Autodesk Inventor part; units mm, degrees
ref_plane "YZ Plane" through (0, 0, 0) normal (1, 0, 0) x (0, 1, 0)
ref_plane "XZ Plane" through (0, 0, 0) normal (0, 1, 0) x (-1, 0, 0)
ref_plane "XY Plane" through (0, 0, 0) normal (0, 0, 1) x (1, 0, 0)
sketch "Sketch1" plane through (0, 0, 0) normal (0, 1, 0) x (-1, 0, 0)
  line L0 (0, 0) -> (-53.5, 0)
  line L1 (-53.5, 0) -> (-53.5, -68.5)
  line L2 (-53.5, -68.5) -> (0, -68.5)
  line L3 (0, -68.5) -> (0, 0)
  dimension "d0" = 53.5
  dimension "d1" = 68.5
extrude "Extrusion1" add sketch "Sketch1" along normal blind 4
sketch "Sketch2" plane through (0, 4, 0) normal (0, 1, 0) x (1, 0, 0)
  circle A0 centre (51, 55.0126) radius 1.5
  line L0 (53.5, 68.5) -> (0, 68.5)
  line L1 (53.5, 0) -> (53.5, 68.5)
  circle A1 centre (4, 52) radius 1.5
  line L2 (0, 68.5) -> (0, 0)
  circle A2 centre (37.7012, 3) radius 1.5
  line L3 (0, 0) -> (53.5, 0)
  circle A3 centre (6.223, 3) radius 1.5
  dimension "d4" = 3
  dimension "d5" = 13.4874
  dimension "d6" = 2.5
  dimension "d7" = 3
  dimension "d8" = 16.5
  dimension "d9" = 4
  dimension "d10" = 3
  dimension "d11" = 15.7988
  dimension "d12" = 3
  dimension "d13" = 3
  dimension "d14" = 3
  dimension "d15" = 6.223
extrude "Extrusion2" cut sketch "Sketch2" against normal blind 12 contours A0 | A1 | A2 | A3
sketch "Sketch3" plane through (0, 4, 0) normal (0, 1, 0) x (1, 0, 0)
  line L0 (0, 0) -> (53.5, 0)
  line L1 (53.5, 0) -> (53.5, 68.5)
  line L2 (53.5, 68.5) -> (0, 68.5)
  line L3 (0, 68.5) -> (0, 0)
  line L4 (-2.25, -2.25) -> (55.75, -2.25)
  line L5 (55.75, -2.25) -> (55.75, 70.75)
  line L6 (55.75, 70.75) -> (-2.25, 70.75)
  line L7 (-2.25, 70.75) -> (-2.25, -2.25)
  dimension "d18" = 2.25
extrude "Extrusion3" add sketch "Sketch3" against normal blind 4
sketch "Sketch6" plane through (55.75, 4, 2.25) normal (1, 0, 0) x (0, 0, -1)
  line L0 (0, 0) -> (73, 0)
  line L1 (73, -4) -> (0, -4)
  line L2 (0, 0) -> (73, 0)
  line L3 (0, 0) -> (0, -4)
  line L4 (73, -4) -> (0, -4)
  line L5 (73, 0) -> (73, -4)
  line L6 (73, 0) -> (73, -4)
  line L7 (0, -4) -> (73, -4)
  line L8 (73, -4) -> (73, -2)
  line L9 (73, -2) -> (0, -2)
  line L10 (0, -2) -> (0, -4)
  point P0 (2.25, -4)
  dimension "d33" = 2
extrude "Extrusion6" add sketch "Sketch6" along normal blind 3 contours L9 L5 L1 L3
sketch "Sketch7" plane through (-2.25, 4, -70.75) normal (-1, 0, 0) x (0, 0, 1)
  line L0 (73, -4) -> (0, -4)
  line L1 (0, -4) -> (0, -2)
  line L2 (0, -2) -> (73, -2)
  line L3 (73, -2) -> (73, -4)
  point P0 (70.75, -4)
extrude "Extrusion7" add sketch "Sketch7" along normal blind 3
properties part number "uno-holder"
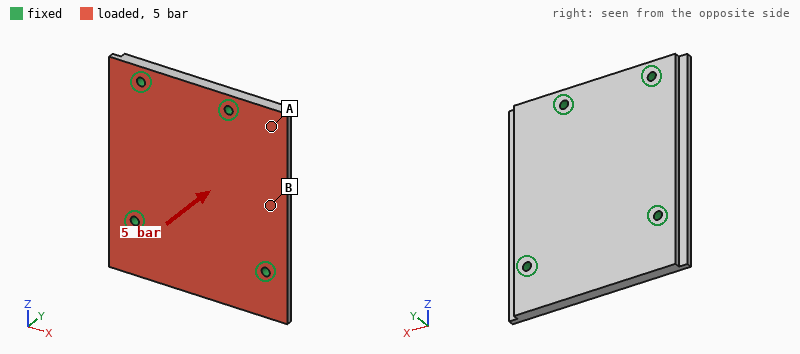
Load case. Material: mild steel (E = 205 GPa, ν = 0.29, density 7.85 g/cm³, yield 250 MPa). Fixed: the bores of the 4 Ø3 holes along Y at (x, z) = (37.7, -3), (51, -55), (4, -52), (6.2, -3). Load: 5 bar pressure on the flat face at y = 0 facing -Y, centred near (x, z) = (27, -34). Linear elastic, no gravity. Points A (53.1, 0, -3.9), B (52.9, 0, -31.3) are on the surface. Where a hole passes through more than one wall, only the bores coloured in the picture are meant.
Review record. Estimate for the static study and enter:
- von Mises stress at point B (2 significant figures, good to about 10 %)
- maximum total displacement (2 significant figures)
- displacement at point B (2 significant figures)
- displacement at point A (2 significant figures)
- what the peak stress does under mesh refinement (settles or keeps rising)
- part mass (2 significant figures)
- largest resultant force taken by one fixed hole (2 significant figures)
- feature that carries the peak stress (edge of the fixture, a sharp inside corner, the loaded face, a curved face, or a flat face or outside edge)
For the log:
29 MPa
21 µm
17 µm
9.2 µm
keeps rising
140 g
700 N
edge of the fixture
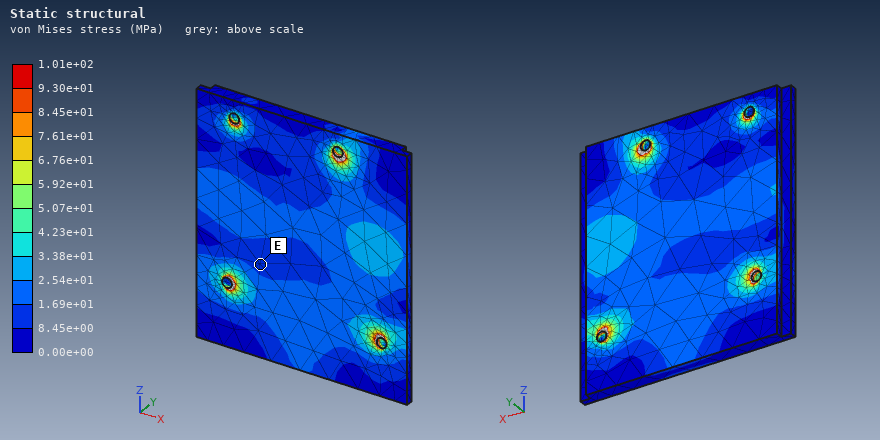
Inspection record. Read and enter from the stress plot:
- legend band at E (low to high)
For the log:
8.45e+00 to 1.69e+01 MPa
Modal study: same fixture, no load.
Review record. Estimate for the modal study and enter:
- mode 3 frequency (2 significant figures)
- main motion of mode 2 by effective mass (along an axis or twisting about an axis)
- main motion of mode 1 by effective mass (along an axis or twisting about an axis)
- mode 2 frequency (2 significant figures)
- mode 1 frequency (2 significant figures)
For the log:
7000 Hz
along Y
along Y
6400 Hz
5700 Hz
